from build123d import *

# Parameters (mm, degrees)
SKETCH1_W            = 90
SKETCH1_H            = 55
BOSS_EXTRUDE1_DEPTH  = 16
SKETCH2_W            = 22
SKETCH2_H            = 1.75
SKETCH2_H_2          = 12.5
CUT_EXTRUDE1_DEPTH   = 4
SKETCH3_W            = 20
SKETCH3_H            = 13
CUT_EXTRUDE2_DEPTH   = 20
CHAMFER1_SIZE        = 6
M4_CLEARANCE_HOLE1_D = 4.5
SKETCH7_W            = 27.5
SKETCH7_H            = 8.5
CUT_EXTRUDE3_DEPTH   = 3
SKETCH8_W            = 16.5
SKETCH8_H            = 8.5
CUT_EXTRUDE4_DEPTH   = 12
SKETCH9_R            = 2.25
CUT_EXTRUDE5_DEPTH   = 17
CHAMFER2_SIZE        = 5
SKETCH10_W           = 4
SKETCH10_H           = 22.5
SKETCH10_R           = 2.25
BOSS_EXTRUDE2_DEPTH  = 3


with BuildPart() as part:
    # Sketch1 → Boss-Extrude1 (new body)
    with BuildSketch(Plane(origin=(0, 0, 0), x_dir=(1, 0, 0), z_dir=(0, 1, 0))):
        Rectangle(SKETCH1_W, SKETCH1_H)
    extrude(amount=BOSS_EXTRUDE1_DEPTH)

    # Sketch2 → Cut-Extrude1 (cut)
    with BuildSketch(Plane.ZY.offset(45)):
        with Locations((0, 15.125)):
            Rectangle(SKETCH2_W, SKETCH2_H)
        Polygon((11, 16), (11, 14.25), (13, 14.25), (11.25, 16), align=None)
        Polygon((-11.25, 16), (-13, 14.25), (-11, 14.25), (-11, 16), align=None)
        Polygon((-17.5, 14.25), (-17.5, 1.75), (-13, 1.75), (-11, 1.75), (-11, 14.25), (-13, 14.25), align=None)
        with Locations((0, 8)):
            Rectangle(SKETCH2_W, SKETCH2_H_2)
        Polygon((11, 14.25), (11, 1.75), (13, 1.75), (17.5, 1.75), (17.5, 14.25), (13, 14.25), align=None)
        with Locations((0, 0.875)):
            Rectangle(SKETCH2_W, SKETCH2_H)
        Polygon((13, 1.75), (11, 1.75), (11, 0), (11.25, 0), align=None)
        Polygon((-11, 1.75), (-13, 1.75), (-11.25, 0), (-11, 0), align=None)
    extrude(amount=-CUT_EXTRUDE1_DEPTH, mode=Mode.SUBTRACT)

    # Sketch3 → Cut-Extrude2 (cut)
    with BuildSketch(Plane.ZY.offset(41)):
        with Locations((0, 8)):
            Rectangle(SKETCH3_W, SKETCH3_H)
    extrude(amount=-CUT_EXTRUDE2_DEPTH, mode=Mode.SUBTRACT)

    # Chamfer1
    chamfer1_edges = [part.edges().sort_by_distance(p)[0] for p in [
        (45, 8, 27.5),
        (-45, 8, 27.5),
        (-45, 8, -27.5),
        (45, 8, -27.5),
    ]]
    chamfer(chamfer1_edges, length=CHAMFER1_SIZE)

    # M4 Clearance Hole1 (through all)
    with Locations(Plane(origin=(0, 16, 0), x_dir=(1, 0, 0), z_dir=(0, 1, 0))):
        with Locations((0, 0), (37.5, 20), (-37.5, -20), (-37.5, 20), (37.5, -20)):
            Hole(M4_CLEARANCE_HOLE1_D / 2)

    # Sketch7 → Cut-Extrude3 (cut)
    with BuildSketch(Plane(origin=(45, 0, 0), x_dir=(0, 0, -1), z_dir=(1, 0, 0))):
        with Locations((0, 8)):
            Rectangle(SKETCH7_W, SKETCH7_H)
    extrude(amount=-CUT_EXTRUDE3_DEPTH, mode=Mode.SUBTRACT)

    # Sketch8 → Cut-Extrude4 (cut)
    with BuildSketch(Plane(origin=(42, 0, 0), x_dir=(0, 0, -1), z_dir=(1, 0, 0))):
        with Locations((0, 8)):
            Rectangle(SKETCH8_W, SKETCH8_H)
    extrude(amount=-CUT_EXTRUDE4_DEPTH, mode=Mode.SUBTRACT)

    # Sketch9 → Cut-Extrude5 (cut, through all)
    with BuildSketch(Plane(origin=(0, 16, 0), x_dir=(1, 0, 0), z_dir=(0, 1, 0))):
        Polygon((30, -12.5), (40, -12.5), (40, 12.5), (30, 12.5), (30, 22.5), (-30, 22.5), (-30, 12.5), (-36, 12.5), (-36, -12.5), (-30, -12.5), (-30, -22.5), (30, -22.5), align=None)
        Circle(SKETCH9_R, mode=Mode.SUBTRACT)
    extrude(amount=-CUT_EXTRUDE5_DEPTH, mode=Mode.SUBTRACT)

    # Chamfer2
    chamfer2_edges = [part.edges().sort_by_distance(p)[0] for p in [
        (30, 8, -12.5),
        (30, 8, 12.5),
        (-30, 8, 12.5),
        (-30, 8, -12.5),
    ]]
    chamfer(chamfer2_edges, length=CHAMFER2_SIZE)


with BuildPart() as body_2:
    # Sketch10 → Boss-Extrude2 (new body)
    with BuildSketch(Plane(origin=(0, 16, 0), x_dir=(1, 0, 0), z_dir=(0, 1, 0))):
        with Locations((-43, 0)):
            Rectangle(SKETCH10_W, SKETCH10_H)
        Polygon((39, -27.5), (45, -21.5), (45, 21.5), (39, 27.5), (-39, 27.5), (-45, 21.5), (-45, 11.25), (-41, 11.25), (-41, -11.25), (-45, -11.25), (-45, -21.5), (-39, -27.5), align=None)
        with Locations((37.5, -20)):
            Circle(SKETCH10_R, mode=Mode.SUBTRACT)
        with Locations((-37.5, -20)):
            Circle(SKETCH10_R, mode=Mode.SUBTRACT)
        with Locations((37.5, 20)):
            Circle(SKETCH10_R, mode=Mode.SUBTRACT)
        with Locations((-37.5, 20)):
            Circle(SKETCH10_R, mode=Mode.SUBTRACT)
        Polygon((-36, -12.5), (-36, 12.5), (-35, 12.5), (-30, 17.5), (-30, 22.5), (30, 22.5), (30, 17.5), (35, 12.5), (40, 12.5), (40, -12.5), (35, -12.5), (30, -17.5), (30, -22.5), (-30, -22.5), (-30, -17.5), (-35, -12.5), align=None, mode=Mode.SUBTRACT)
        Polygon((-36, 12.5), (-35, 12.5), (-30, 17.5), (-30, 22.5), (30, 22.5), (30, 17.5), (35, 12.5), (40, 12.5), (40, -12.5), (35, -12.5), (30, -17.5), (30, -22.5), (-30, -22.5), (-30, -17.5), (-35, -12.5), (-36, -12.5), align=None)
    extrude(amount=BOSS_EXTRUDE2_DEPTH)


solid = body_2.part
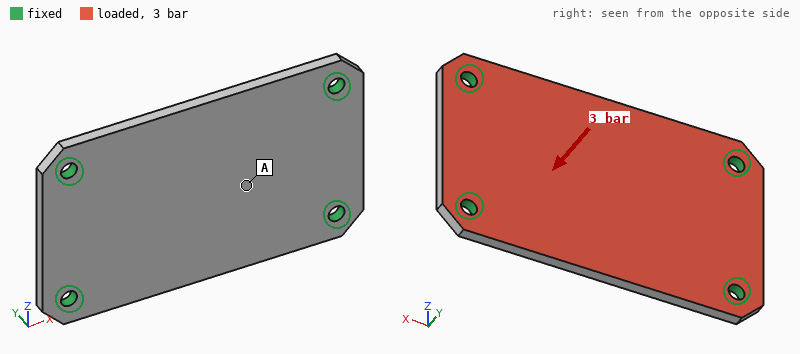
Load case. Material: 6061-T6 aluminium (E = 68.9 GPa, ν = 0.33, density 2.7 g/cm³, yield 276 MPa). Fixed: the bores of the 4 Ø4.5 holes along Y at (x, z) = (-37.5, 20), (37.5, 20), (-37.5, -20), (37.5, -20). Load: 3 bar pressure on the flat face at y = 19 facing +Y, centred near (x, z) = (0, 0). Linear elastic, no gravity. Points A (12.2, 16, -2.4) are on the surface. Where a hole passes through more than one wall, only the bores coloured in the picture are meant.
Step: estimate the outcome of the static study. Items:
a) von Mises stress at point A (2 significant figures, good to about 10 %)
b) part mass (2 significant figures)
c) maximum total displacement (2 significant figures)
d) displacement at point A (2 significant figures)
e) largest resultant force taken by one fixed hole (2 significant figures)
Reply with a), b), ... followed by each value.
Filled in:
a) 30 MPa
b) 39 g
c) 0.18 mm
d) 0.15 mm
e) 360 N
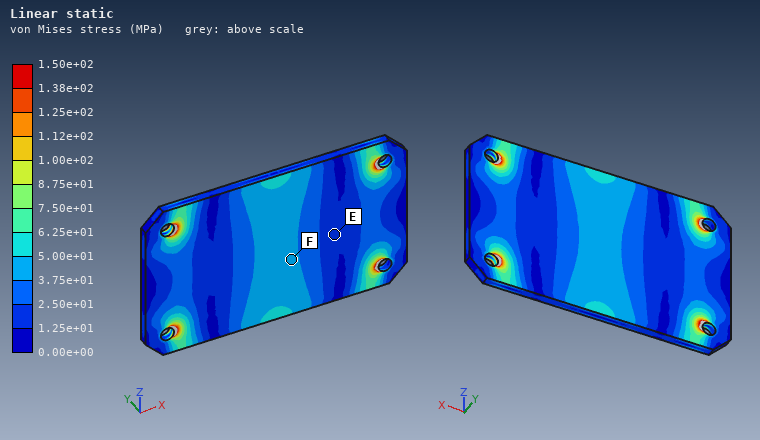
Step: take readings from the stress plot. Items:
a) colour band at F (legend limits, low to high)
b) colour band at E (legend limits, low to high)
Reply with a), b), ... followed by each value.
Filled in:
a) 3.75e+01 to 5.00e+01 MPa
b) 1.25e+01 to 2.50e+01 MPa
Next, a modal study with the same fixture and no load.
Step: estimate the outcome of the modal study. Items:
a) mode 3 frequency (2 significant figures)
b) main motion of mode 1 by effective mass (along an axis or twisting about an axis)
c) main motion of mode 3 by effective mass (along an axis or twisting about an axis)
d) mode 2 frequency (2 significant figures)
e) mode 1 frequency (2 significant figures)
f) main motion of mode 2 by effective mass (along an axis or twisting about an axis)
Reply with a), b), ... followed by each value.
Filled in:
a) 6900 Hz
b) along Y
c) twisting about Z
d) 3800 Hz
e) 2600 Hz
f) twisting about X
